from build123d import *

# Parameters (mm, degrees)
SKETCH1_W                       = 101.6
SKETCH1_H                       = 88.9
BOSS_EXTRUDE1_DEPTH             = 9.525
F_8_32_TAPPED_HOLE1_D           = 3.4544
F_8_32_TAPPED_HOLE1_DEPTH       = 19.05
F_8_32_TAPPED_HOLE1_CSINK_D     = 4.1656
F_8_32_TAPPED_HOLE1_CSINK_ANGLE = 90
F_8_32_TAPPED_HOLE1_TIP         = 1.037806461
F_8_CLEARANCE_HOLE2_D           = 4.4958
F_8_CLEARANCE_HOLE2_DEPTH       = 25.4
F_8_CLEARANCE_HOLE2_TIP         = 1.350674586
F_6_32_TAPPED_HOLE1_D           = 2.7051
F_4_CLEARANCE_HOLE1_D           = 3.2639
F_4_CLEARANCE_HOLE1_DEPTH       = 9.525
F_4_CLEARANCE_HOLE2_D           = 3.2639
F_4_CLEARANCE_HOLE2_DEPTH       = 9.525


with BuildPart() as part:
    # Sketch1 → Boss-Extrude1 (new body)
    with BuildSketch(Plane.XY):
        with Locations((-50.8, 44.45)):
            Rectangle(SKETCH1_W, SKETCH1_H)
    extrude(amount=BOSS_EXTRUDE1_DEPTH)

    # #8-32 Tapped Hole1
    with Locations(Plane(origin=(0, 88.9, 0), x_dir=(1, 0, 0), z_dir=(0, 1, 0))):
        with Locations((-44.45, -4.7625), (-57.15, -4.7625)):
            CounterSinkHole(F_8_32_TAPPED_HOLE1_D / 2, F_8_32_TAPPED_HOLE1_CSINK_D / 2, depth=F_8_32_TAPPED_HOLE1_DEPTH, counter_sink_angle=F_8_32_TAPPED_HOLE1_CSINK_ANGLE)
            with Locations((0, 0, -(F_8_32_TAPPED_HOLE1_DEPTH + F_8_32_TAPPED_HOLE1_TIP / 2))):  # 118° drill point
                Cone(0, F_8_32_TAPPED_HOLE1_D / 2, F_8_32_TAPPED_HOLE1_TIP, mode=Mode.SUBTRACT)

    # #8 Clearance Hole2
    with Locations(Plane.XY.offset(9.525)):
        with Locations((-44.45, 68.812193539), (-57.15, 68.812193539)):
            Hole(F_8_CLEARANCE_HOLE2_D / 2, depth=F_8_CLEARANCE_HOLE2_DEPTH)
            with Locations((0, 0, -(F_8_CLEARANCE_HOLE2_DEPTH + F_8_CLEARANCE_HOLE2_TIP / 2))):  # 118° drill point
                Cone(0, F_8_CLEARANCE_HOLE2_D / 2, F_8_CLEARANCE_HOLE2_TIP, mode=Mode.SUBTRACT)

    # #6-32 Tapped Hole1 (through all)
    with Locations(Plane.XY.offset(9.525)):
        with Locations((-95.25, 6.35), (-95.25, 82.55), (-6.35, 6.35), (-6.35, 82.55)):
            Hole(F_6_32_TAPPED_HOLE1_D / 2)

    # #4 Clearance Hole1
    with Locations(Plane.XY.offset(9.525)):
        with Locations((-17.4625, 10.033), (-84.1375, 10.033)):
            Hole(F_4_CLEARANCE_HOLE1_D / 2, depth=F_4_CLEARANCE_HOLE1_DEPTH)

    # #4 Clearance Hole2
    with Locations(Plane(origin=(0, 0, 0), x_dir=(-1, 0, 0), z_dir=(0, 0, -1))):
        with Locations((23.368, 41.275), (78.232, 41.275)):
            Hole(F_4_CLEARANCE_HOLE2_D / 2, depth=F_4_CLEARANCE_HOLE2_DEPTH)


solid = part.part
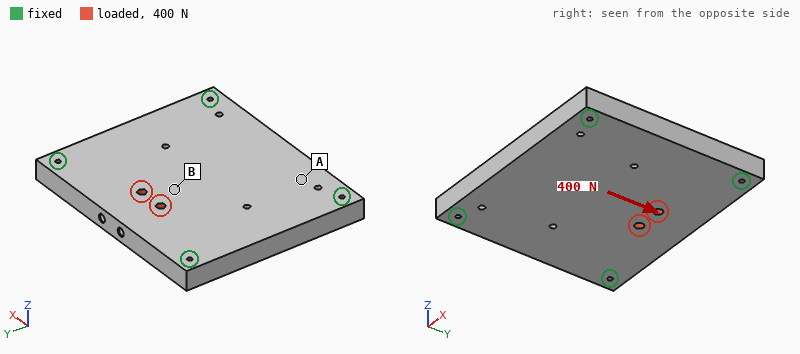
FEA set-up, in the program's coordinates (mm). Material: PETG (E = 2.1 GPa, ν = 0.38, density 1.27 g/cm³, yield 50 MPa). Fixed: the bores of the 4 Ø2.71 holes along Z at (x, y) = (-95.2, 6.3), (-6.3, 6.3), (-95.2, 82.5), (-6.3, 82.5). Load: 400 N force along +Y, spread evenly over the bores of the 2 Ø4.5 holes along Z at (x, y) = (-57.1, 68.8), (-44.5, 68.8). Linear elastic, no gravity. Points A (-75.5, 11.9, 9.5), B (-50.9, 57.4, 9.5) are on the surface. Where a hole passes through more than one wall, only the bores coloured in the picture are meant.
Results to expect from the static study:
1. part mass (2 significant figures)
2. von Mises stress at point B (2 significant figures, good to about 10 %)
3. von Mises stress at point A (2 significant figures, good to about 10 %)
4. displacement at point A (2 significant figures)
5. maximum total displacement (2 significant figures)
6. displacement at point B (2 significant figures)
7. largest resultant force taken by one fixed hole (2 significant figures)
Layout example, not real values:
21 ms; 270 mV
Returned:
110 g; 0.97 MPa; 0.32 MPa; 10 µm; 31 µm; 23 µm; 120 N
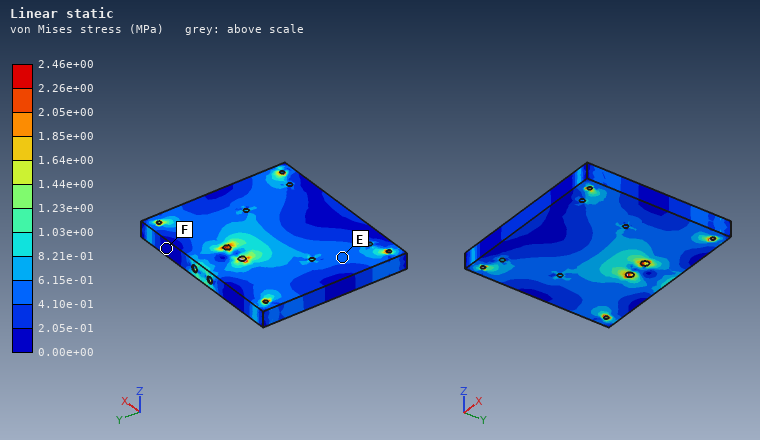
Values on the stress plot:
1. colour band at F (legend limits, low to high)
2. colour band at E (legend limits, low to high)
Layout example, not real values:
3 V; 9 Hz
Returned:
0.00e+00 to 2.05e-01 MPa; 4.10e-01 to 6.15e-01 MPa
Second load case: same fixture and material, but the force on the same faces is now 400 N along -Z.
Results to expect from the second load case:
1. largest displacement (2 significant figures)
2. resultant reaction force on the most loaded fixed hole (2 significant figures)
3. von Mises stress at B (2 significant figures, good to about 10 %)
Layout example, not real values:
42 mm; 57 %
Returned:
0.34 mm; 170 N; 4.4 MPa
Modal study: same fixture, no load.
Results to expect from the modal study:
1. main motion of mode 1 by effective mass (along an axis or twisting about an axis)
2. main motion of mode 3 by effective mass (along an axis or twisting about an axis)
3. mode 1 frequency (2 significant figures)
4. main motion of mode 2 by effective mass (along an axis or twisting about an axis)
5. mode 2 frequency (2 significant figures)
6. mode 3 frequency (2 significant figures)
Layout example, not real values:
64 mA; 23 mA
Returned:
along Z; twisting about Y; 970 Hz; twisting about X; 1600 Hz; 1800 Hz
